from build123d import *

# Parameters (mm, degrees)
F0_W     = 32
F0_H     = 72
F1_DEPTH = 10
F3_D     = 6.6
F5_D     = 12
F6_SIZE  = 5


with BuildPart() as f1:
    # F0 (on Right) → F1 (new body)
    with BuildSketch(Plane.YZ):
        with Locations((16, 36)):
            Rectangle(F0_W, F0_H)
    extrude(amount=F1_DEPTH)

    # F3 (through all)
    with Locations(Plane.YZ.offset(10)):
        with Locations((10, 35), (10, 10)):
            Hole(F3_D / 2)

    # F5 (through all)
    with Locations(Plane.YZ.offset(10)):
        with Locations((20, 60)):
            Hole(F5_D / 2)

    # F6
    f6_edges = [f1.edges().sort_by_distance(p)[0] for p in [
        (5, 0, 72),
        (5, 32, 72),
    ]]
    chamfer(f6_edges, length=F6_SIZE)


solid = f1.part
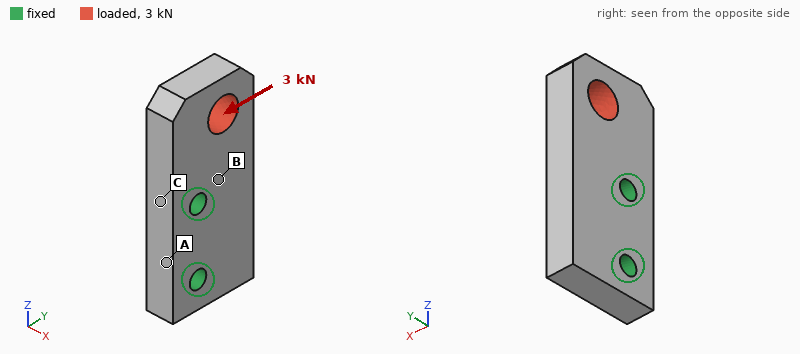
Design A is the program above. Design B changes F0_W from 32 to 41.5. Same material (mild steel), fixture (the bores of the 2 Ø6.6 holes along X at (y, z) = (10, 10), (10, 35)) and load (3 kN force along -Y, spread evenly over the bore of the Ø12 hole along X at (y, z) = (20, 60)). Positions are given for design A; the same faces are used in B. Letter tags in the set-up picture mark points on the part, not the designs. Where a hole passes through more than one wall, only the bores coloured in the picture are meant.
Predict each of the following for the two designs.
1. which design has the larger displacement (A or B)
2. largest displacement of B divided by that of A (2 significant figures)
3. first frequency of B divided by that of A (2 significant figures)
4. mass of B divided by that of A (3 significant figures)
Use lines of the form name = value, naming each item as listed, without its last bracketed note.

which design has the larger displacement = A
largest displacement of B divided by that of A = 0.70
first frequency of B divided by that of A = 0.92
mass of B divided by that of A = 1.33
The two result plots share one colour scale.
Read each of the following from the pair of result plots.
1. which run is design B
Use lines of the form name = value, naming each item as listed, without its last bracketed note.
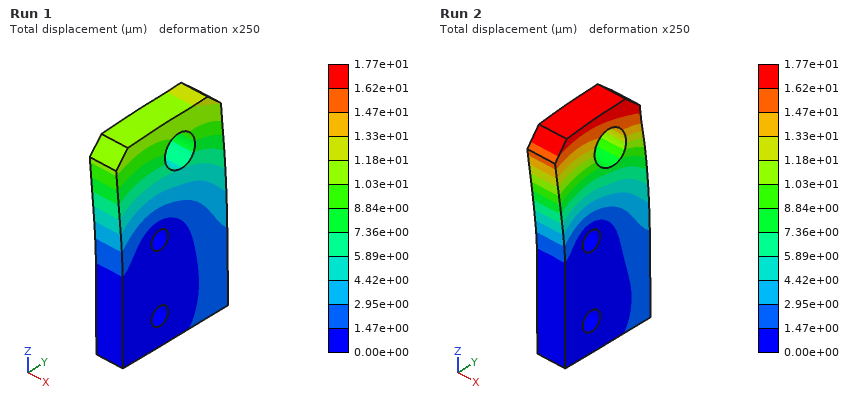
which run is design B = Run 1
